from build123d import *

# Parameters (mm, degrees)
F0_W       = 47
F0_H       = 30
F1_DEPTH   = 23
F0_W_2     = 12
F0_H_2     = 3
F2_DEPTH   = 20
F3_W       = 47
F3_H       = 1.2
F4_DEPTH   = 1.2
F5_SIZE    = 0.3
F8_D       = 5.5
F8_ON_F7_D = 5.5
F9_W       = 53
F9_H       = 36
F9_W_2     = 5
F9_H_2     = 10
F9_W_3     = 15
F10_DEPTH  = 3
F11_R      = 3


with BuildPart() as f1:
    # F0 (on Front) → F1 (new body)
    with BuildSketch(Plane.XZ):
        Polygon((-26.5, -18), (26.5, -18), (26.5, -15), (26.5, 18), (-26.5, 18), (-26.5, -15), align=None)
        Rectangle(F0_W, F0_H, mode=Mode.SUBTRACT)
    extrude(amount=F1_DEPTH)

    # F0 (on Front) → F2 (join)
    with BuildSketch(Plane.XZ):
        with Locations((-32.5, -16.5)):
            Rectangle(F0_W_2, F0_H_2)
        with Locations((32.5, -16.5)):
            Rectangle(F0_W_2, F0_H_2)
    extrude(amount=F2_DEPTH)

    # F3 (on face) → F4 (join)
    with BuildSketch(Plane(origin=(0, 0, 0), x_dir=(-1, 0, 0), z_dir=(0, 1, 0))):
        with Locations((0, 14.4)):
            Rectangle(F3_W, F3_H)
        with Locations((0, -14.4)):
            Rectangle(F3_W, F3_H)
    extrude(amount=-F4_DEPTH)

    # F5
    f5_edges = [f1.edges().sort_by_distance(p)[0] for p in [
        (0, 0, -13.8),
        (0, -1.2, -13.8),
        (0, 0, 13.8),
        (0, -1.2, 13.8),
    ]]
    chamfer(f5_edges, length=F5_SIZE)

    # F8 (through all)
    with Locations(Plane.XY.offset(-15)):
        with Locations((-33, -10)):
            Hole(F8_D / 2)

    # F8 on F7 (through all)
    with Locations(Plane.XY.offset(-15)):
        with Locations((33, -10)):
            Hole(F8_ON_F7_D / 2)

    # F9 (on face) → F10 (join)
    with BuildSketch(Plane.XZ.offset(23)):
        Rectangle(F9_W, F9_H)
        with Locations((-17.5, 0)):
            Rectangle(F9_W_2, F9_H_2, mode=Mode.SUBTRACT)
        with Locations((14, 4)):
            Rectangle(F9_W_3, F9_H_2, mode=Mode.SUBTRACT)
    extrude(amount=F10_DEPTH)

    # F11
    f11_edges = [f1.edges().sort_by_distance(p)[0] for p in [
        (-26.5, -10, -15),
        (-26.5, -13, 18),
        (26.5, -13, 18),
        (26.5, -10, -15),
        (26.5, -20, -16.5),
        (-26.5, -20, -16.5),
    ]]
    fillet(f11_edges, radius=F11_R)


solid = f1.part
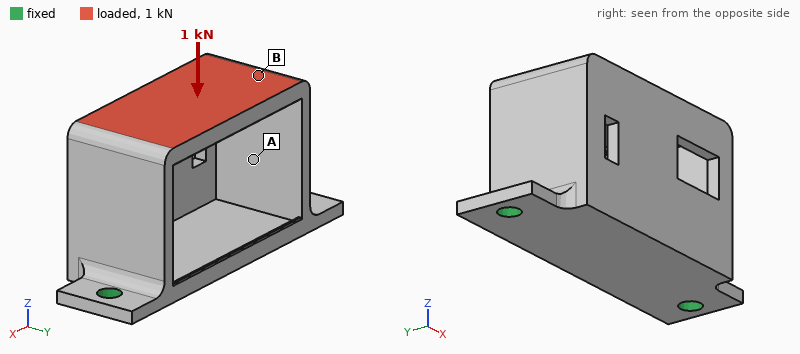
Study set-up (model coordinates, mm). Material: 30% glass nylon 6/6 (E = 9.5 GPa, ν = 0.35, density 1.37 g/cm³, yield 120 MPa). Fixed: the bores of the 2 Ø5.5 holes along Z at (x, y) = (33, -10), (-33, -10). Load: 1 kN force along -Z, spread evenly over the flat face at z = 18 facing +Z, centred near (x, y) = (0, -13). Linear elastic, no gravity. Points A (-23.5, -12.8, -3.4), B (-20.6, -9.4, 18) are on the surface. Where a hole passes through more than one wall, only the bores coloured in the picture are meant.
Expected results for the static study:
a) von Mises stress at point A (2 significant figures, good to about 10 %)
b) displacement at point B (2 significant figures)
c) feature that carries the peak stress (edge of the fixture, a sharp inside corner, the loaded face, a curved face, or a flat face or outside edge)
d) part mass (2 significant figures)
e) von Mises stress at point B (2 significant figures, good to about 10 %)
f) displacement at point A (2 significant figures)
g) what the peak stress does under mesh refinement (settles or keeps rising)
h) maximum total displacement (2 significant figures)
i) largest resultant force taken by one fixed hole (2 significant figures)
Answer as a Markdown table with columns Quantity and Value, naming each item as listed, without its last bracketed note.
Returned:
| Quantity | Value |
|---|---|
| von Mises stress at point A | 11 MPa |
| displacement at point B | 0.30 mm |
| feature that carries the peak stress | edge of the fixture |
| part mass | 25 g |
| von Mises stress at point B | 30 MPa |
| displacement at point A | 0.13 mm |
| what the peak stress does under mesh refinement | keeps rising |
| maximum total displacement | 0.72 mm |
| largest resultant force taken by one fixed hole | 520 N |
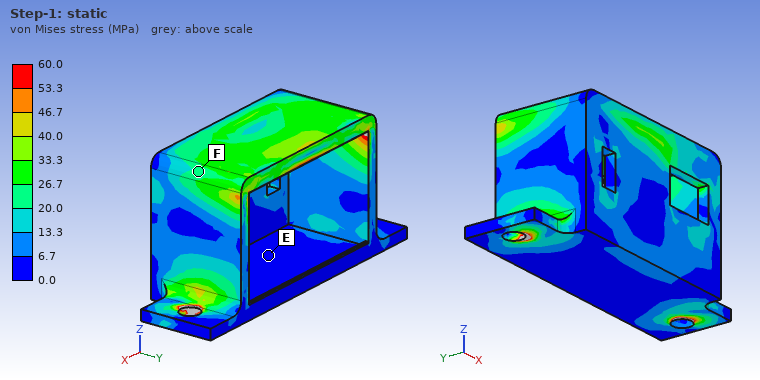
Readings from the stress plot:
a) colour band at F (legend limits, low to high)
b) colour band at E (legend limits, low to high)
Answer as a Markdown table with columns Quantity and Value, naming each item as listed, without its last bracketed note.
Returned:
| Quantity | Value |
|---|---|
| colour band at F | 20.0 to 26.7 MPa |
| colour band at E | 0.0 to 6.7 MPa |
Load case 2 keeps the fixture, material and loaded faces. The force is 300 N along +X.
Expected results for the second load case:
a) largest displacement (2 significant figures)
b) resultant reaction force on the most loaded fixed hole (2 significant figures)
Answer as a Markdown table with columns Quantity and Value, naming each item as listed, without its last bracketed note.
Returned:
| Quantity | Value |
|---|---|
| largest displacement | 0.59 mm |
| resultant reaction force on the most loaded fixed hole | 230 N |
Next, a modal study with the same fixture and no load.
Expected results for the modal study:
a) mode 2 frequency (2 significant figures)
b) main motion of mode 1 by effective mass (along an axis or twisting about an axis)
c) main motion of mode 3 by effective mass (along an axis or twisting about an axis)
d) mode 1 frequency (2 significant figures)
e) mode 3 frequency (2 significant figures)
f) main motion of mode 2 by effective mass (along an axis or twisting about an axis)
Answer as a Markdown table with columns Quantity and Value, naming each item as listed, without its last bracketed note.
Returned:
| Quantity | Value |
|---|---|
| mode 2 frequency | 1300 Hz |
| main motion of mode 1 by effective mass | along Y |
| main motion of mode 3 by effective mass | along Z |
| mode 1 frequency | 850 Hz |
| mode 3 frequency | 2900 Hz |
| main motion of mode 2 by effective mass | along X |
